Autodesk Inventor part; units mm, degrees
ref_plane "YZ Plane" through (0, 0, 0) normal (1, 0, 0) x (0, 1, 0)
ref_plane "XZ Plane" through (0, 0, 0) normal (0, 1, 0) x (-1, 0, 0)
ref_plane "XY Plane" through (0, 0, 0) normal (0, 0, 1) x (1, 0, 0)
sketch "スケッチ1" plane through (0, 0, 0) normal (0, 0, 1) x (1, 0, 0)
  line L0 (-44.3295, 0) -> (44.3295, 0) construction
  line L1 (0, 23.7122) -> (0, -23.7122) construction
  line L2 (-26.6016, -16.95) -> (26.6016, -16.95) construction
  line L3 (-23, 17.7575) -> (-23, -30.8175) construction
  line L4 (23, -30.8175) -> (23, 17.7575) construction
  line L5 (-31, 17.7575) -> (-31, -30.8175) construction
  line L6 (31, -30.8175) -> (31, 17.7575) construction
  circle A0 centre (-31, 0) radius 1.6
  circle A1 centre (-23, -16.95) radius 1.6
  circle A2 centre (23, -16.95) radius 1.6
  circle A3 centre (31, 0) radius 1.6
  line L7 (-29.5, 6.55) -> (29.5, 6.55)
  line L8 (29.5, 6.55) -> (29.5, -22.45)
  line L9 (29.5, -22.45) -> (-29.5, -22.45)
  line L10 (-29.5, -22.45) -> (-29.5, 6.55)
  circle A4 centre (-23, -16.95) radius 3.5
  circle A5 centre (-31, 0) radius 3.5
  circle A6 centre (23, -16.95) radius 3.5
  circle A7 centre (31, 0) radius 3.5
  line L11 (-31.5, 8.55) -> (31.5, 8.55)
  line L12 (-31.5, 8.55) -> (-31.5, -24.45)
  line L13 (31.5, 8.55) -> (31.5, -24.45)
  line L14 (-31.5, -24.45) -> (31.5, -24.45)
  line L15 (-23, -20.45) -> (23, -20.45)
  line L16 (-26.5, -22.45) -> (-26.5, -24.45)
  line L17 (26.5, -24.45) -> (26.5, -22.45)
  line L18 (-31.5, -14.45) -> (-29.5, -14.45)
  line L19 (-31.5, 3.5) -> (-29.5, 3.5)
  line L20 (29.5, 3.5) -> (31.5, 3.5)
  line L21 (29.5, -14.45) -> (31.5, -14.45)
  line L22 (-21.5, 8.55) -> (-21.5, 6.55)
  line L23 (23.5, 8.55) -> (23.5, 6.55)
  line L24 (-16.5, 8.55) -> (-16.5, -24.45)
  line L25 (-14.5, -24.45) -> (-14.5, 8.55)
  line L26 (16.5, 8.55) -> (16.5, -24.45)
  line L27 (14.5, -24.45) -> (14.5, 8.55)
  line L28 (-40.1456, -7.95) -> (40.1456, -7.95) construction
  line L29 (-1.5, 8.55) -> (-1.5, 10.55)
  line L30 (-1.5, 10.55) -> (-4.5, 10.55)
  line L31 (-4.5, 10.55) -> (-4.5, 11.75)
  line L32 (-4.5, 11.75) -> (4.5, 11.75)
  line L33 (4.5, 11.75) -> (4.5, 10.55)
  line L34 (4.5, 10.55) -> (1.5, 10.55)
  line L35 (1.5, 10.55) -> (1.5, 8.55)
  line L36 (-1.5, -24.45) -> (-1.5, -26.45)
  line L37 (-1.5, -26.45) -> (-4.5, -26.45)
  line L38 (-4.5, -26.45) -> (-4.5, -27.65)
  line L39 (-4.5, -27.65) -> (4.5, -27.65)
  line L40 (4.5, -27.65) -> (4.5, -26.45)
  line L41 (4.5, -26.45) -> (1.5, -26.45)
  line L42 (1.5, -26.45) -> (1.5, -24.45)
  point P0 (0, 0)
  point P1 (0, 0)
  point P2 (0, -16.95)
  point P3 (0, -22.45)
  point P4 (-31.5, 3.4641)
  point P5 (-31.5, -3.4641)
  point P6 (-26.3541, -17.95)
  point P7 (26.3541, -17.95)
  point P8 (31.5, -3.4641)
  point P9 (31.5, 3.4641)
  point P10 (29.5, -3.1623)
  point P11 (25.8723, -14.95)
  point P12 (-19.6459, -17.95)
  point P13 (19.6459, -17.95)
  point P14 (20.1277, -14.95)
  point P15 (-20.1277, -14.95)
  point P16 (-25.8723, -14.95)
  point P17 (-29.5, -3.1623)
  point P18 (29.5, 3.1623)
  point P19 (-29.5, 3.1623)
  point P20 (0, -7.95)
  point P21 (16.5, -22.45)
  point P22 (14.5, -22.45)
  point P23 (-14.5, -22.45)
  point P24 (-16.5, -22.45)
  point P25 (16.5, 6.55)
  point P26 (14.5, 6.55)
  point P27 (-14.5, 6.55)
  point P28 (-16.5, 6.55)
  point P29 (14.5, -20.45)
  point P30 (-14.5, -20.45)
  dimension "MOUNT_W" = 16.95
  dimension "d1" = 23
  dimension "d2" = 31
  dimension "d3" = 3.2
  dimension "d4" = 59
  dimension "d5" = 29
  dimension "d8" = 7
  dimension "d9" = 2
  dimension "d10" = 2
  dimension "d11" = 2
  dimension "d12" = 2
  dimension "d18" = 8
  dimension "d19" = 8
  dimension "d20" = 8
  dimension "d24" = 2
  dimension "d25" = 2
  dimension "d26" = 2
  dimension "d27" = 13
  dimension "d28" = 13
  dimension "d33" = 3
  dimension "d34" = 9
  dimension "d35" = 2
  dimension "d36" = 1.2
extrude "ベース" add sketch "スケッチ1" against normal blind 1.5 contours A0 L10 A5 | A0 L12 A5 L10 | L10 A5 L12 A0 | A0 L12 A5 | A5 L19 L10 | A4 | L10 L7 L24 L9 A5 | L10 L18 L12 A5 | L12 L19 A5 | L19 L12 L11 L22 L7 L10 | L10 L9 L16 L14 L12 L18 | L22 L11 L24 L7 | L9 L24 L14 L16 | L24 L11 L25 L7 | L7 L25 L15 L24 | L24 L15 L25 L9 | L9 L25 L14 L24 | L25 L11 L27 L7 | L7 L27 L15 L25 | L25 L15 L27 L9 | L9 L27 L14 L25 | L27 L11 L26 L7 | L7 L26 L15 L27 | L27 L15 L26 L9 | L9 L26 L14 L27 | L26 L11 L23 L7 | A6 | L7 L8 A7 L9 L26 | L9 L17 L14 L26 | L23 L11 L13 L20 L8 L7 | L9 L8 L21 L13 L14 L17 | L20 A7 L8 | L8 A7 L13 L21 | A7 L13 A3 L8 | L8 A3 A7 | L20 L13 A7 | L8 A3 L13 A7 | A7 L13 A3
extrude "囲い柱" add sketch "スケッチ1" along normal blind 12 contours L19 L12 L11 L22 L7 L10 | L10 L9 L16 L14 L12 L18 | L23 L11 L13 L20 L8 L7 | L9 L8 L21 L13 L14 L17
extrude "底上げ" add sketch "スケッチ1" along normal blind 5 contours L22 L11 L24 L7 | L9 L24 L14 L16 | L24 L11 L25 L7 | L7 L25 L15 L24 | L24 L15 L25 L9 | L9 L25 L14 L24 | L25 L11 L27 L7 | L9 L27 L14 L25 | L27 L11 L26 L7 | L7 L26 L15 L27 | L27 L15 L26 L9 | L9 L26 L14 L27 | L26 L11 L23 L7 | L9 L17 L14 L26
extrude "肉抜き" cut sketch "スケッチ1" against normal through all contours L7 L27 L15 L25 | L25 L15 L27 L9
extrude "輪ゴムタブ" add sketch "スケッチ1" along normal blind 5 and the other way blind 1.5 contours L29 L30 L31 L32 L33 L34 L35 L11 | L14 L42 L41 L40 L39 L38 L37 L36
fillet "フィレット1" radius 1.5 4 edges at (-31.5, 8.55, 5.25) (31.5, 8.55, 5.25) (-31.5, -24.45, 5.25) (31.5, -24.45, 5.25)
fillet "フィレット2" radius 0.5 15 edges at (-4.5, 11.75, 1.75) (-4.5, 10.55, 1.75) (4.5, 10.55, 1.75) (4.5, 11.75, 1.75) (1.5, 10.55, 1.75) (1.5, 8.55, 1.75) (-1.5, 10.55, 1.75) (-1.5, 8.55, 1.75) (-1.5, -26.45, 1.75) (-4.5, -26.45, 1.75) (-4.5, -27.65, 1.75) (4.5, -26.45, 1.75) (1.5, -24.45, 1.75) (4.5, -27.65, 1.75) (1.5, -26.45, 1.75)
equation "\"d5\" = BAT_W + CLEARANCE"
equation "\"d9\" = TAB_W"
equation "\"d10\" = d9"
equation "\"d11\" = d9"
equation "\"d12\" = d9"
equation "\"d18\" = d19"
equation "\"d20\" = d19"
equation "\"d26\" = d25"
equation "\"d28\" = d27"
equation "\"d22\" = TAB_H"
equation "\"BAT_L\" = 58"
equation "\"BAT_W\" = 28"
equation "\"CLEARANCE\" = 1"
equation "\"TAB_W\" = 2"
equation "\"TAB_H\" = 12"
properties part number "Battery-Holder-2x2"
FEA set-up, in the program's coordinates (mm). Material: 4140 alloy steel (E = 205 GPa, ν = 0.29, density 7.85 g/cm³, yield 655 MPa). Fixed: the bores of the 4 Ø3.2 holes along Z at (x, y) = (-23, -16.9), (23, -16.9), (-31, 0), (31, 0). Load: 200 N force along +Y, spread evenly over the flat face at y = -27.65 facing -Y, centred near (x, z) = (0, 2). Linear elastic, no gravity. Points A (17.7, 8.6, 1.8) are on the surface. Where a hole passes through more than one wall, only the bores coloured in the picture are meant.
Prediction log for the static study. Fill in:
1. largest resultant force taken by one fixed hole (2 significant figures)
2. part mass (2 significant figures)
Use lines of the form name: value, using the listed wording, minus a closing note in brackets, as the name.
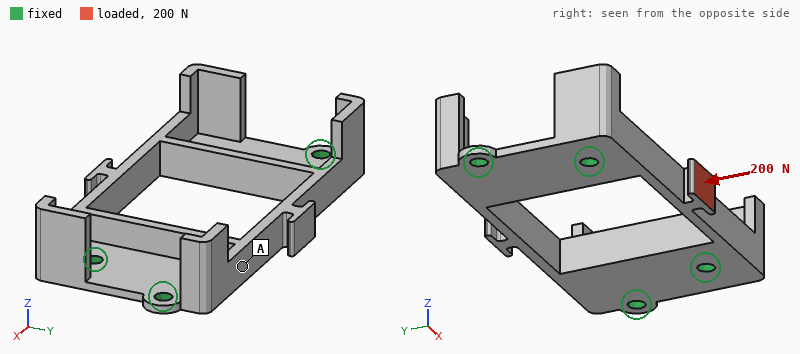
largest resultant force taken by one fixed hole: 83 N
part mass: 38 g
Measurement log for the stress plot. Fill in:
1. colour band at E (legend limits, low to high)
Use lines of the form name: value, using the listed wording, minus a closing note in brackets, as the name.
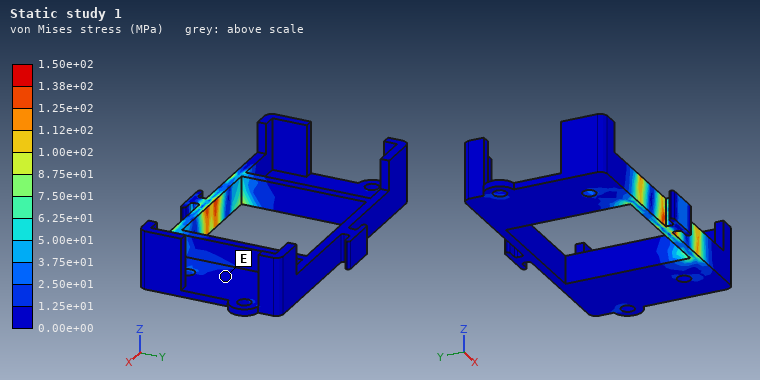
colour band at E: 0.00e+00 to 1.25e+01 MPa
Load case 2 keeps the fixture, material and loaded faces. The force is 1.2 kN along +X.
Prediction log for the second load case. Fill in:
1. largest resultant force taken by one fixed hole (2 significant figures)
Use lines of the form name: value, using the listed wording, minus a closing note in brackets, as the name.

largest resultant force taken by one fixed hole: 640 N
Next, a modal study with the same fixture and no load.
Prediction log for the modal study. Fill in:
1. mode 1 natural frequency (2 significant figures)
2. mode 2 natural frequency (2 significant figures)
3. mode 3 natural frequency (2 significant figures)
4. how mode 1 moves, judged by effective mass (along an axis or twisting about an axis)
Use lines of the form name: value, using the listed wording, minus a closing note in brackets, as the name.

mode 1 natural frequency: 3900 Hz
mode 2 natural frequency: 5900 Hz
mode 3 natural frequency: 7000 Hz
how mode 1 moves, judged by effective mass: along Z
